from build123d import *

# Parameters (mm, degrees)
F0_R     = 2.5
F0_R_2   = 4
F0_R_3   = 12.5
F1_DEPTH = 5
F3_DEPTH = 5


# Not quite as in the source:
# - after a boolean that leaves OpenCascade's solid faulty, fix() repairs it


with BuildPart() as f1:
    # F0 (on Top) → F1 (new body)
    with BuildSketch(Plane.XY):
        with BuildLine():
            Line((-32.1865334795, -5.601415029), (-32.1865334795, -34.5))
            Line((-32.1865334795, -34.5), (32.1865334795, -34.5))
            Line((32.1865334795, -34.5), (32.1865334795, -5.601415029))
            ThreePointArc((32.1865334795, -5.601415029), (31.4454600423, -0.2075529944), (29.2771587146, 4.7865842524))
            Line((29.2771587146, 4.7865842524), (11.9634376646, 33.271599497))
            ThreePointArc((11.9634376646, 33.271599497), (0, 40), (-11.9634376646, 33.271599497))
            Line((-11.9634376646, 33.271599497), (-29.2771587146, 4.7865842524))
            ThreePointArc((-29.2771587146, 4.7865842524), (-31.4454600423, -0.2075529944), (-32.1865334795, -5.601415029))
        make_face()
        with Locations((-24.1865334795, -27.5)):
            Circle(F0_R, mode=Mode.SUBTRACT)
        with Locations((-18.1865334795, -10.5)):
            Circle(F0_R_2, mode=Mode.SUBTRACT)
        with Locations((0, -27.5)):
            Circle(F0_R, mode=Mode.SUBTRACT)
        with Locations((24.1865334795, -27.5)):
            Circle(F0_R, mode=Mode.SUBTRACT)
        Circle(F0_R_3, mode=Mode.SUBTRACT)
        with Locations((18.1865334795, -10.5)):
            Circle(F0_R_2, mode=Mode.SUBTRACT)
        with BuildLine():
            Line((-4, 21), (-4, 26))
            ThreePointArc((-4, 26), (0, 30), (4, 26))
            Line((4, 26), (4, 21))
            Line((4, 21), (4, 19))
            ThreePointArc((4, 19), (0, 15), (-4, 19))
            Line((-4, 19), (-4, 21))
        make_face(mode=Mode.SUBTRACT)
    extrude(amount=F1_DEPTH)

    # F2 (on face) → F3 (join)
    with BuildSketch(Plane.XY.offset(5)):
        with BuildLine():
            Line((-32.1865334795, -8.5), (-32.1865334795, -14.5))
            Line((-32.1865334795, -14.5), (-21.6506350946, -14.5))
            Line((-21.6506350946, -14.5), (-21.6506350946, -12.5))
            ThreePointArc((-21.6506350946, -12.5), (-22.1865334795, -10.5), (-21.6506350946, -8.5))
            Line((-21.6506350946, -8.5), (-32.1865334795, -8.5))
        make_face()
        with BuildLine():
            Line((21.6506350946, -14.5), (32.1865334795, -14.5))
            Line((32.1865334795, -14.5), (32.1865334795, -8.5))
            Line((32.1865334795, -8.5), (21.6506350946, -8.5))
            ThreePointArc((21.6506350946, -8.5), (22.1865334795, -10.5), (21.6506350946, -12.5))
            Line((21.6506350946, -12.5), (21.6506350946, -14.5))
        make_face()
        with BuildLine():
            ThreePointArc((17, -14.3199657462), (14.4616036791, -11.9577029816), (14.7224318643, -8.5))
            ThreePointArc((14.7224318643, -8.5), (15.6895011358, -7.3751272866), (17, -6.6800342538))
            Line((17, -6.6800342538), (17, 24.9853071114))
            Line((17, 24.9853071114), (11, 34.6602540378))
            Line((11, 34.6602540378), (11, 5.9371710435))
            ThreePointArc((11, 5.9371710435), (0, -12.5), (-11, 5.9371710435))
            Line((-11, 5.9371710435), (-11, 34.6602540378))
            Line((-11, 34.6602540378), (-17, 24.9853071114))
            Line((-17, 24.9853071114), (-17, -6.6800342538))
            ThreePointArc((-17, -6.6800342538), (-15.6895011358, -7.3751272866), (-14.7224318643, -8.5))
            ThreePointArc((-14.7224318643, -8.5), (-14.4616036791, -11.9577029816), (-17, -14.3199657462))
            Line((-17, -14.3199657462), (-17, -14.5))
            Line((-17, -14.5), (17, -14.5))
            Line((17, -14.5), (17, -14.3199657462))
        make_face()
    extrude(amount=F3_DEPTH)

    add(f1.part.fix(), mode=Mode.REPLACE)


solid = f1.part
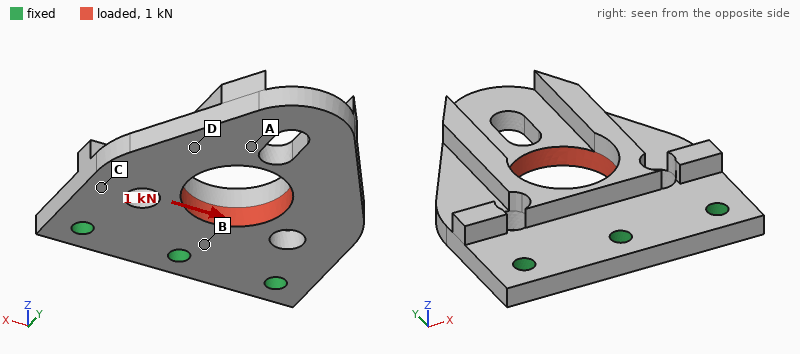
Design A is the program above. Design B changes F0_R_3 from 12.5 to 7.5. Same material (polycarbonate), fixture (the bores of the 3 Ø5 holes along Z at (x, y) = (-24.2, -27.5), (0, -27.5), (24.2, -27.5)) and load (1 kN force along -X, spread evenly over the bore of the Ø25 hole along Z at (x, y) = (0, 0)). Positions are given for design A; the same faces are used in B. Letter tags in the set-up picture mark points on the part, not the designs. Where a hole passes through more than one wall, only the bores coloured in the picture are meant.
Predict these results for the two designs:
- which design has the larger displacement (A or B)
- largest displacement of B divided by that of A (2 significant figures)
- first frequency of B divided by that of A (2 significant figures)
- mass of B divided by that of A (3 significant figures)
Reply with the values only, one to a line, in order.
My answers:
A
0.70
1.0
1.08
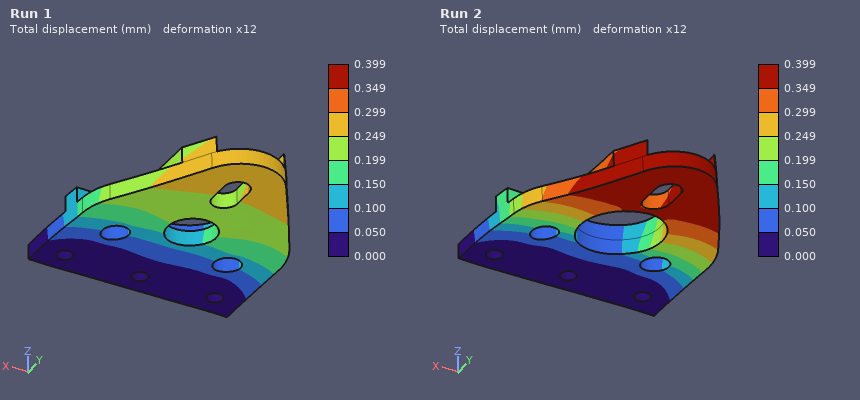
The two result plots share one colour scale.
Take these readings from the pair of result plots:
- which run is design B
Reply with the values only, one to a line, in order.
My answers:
Run 1
